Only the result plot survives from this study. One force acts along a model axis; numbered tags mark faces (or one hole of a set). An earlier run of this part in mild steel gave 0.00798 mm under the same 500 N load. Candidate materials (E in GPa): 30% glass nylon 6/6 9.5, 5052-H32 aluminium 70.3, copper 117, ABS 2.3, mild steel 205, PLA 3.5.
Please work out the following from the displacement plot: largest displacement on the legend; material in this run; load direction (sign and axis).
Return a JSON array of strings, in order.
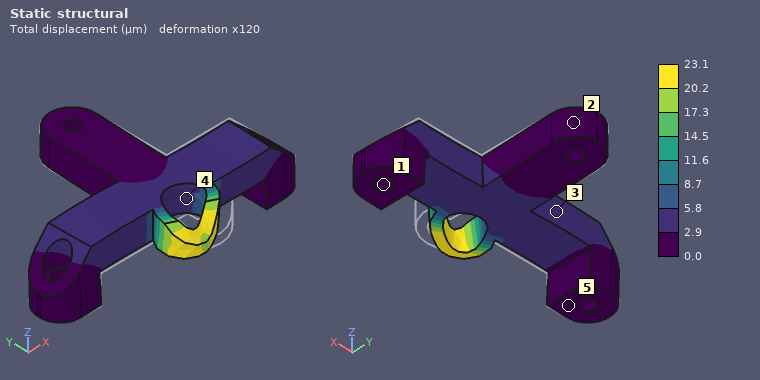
["23.1 µm", "5052-H32 aluminium", "-X"]
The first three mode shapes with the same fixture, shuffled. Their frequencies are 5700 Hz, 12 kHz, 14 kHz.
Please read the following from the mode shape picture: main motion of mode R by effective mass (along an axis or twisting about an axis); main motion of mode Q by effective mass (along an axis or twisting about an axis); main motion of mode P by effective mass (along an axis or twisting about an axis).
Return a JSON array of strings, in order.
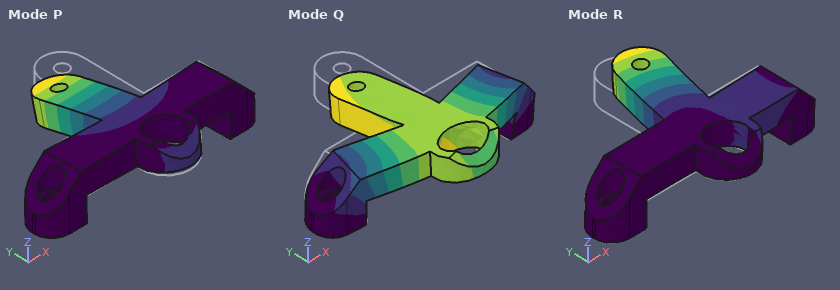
["along X", "along Y", "along Z"]
